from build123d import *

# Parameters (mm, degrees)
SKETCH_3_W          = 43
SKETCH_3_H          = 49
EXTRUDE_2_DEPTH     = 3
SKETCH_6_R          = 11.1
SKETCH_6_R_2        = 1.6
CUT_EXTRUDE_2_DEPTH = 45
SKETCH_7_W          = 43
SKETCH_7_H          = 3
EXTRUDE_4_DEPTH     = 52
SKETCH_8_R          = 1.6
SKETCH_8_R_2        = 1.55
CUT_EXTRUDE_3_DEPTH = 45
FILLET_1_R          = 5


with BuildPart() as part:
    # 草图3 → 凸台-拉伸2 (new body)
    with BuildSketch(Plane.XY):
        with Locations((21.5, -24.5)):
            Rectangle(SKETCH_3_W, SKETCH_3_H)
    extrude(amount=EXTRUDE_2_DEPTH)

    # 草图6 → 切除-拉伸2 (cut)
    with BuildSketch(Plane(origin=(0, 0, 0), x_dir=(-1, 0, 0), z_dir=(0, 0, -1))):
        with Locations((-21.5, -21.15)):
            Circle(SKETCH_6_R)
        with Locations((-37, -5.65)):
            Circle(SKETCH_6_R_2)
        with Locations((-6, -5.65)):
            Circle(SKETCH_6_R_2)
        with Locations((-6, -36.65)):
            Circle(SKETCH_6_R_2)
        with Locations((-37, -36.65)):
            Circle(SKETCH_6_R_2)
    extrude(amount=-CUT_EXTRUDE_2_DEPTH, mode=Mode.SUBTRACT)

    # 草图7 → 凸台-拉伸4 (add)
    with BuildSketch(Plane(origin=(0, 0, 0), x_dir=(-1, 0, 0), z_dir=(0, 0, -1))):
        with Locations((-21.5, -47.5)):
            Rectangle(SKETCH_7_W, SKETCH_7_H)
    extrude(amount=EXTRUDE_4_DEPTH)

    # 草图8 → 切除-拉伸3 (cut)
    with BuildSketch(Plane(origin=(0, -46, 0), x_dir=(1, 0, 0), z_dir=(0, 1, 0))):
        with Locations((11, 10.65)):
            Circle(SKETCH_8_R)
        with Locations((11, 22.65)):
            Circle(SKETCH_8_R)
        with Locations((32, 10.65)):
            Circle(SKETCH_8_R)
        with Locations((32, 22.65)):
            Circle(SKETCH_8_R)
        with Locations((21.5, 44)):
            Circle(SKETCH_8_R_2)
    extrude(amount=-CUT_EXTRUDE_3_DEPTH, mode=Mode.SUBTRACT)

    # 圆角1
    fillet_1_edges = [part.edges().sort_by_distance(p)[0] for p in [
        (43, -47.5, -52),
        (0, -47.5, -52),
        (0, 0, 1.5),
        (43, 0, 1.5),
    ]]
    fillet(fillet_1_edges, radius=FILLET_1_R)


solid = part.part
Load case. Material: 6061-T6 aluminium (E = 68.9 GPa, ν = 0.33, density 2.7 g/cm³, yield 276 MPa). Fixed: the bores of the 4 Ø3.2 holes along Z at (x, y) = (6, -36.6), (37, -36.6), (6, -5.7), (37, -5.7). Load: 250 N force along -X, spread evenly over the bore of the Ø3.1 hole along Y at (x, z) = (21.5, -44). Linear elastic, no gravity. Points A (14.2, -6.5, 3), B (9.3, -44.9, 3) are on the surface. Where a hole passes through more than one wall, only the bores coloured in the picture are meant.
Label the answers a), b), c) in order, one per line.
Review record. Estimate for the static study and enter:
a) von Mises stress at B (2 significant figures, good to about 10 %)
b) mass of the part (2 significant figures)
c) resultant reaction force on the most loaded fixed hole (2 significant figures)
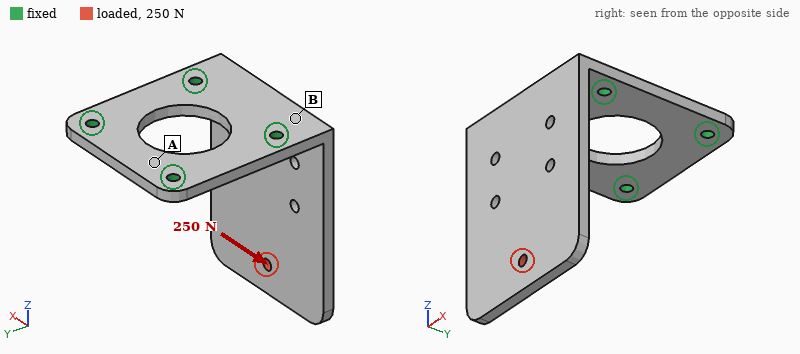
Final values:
a) 37 MPa
b) 31 g
c) 390 N
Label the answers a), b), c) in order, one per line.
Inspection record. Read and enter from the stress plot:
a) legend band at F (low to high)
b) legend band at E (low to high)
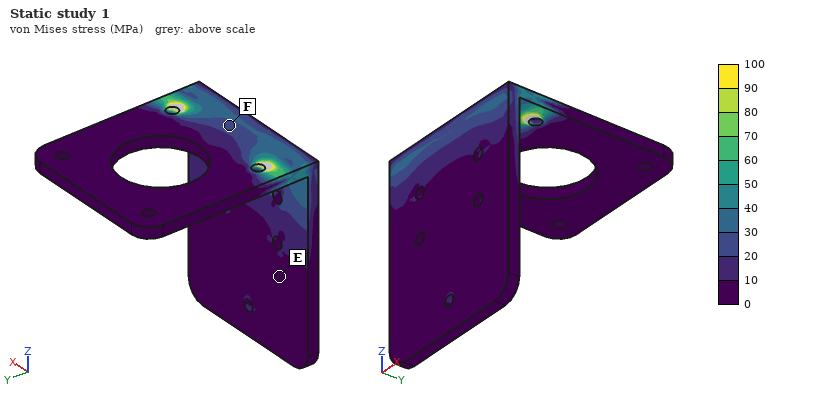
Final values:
a) 20 to 30 MPa
b) 0 to 10 MPa
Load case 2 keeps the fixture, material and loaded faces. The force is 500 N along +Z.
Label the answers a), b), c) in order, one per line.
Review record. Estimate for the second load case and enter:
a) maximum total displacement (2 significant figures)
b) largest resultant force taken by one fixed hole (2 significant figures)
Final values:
a) 0.27 mm
b) 260 N
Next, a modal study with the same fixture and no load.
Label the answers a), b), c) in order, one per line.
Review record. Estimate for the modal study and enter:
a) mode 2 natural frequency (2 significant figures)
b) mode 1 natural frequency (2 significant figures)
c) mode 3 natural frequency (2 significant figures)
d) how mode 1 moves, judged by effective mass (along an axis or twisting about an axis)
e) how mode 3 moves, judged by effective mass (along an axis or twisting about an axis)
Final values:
a) 2000 Hz
b) 650 Hz
c) 2800 Hz
d) along Y
e) along X
